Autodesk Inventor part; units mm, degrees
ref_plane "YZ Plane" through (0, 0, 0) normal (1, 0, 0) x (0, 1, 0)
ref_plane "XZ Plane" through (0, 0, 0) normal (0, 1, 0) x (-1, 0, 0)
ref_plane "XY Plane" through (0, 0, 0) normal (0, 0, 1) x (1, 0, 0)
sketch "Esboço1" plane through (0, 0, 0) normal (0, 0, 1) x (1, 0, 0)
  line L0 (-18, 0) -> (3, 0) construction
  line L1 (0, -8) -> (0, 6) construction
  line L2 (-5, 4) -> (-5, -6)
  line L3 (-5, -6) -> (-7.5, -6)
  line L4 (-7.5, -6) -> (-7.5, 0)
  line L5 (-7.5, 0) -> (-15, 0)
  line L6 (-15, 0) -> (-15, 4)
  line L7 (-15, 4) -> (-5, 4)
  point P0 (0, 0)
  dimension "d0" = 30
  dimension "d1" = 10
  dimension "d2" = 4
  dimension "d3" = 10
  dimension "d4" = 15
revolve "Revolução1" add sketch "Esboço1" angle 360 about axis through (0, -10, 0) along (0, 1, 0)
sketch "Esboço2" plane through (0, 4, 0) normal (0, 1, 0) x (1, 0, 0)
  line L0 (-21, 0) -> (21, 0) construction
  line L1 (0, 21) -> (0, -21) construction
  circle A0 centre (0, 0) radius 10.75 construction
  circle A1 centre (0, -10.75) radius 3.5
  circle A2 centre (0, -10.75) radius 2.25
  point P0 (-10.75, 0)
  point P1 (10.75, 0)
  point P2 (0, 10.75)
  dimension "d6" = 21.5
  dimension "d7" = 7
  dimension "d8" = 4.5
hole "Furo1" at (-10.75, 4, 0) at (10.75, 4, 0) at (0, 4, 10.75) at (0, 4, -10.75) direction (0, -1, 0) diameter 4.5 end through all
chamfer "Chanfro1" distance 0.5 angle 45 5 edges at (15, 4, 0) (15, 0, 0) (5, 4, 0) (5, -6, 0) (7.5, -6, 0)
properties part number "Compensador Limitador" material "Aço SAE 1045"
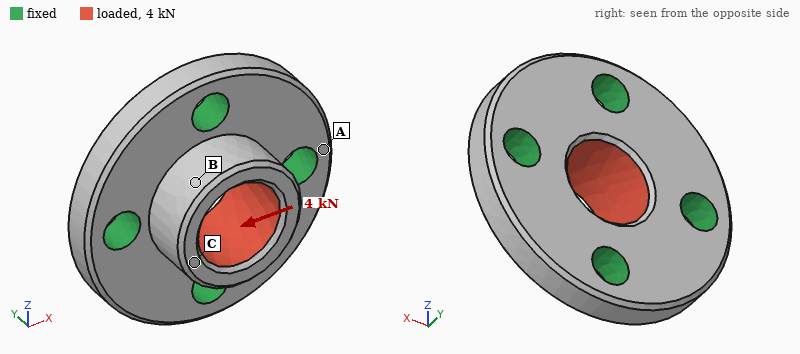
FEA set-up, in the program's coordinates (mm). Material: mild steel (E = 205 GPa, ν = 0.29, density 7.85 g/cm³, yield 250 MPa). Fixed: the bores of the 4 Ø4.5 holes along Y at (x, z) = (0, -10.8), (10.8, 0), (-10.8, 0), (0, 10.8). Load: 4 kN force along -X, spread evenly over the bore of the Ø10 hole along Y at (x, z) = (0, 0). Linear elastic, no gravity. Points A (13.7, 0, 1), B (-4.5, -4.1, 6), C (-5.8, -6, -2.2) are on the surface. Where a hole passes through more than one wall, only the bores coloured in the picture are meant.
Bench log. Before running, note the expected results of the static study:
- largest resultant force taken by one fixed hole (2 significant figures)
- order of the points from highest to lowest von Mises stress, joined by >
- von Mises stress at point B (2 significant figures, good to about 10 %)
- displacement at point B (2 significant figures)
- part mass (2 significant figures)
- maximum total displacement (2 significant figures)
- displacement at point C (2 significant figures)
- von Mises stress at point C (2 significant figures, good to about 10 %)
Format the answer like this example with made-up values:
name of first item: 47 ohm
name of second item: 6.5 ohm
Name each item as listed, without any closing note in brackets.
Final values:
largest resultant force taken by one fixed hole: 1.3 kN
order of the points from highest to lowest von Mises stress, joined by >: C > B > A
von Mises stress at point B: 19 MPa
displacement at point B: 2.8 µm
part mass: 22 g
maximum total displacement: 3.9 µm
displacement at point C: 3.8 µm
von Mises stress at point C: 36 MPa
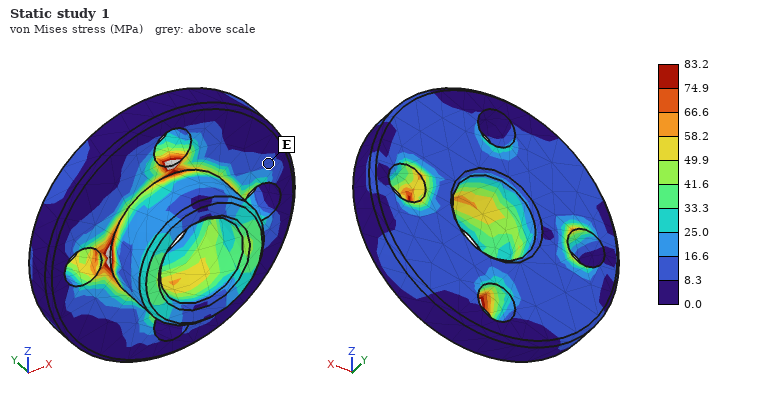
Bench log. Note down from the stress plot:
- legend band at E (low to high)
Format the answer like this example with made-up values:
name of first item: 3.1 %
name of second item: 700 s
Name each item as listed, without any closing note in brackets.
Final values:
legend band at E: 8.3 to 16.6 MPa
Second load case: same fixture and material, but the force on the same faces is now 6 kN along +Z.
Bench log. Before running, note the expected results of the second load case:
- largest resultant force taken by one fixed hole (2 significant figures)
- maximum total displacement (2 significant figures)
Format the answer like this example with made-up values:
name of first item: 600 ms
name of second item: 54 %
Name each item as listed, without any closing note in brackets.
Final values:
largest resultant force taken by one fixed hole: 1.9 kN
maximum total displacement: 5.8 µm
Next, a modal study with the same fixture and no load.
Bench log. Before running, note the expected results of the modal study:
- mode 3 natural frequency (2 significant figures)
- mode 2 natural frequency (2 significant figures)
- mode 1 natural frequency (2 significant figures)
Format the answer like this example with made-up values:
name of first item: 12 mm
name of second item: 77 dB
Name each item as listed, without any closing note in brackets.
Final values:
mode 3 natural frequency: 61 kHz
mode 2 natural frequency: 61 kHz
mode 1 natural frequency: 59 kHz
